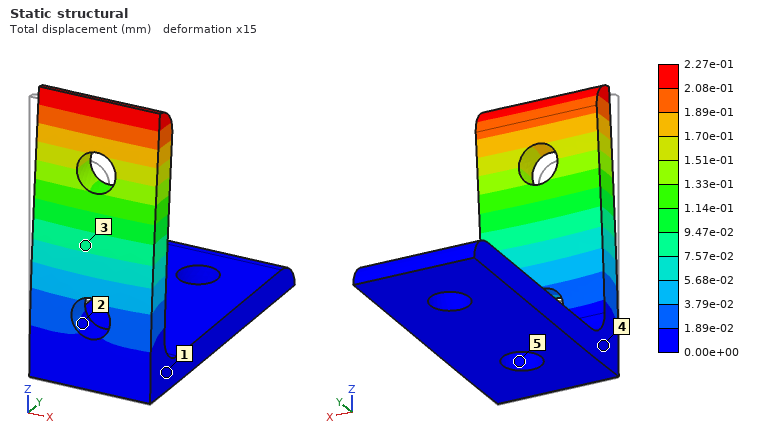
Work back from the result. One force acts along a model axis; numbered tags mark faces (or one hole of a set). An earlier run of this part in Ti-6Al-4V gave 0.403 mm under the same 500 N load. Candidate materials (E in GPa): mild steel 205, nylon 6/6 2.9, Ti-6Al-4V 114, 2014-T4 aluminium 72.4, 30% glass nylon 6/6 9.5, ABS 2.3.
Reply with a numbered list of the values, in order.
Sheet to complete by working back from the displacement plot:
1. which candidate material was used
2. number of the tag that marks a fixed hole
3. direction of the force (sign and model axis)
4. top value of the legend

1. mild steel
2. 5
3. +Y
4. 2.27e-01 mm
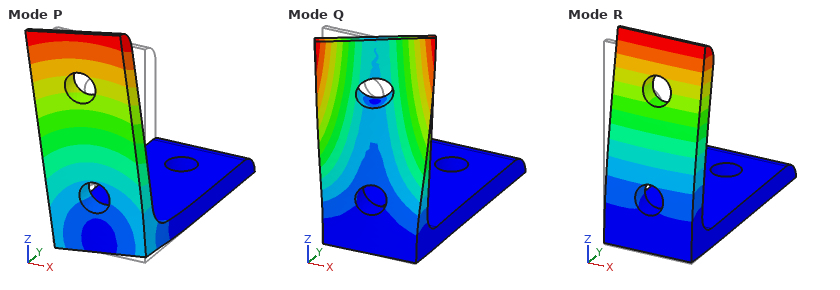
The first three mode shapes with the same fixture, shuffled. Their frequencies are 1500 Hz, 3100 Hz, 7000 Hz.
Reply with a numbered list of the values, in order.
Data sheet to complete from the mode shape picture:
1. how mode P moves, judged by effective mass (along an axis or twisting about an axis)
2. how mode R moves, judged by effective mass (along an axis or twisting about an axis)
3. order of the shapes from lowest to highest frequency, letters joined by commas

1. along X
2. along Y
3. R, P, Q
